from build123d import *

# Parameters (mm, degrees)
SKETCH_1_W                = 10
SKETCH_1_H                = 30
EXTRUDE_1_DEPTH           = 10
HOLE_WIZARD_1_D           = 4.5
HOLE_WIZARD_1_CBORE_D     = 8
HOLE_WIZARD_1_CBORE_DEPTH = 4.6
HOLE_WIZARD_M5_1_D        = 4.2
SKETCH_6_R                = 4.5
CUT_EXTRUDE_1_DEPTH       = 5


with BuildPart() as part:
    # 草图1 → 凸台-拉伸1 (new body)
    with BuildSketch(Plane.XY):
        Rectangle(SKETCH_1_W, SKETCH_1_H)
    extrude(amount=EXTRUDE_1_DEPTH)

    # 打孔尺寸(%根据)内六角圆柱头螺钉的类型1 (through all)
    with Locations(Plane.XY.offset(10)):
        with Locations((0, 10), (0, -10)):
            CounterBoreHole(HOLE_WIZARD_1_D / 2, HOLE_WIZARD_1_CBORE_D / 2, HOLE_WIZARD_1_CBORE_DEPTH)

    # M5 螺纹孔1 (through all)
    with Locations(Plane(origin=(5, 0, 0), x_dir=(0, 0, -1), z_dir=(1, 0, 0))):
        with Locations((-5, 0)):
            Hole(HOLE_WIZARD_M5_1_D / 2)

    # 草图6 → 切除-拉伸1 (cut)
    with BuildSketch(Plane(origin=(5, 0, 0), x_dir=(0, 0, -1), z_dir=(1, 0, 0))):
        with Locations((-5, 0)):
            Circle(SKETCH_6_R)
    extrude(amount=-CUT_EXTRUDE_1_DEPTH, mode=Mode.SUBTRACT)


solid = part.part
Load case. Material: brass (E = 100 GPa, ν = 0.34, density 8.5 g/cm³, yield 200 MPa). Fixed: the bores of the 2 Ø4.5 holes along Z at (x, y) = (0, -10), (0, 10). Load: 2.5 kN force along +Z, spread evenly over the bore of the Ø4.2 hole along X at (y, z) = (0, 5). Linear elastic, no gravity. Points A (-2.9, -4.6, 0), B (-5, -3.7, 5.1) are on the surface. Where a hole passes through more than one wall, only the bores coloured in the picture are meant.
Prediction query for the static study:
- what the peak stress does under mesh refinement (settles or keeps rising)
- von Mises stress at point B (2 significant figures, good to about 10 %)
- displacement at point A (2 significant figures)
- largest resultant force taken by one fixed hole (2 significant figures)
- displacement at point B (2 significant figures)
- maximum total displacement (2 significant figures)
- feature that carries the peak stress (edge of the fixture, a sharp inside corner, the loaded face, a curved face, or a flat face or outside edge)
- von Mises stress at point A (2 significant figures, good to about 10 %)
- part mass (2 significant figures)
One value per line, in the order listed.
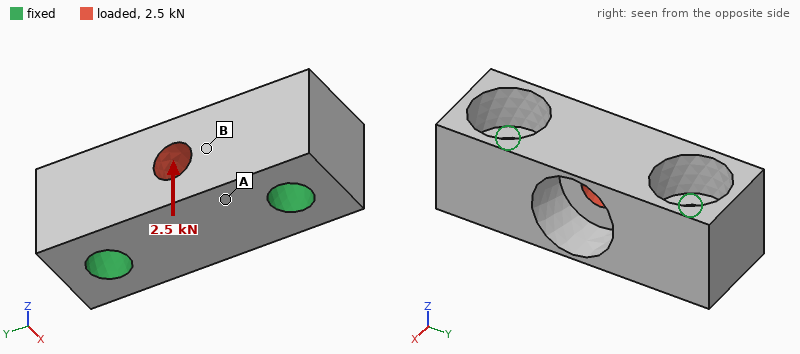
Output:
keeps rising
57 MPa
5.9 µm
1.3 kN
8.0 µm
11 µm
edge of the fixture
20 MPa
17 g
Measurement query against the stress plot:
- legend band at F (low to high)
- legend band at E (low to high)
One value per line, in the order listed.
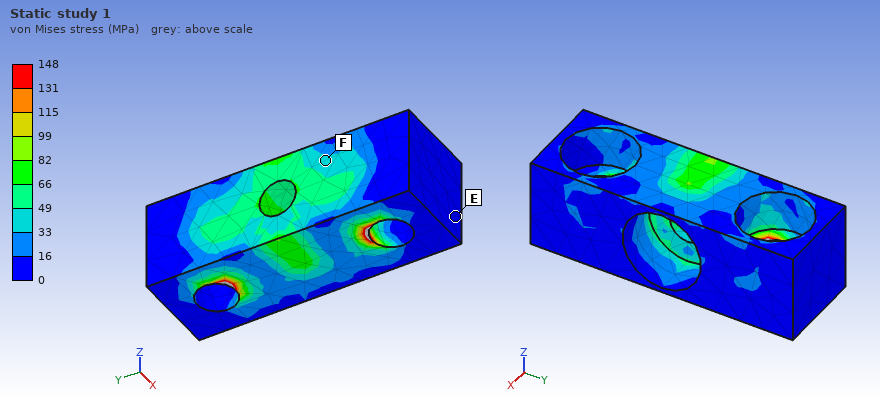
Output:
33 to 49 MPa
0 to 16 MPa
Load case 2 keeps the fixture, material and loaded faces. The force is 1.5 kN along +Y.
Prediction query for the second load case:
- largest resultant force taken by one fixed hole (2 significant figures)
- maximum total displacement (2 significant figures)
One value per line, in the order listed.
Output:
770 N
2.6 µm
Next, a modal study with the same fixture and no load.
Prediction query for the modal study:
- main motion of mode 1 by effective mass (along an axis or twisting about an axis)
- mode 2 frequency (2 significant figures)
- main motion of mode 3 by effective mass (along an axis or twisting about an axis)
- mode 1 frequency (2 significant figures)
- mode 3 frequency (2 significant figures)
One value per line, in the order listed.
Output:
along X
41 kHz
along Z
30 kHz
44 kHz
